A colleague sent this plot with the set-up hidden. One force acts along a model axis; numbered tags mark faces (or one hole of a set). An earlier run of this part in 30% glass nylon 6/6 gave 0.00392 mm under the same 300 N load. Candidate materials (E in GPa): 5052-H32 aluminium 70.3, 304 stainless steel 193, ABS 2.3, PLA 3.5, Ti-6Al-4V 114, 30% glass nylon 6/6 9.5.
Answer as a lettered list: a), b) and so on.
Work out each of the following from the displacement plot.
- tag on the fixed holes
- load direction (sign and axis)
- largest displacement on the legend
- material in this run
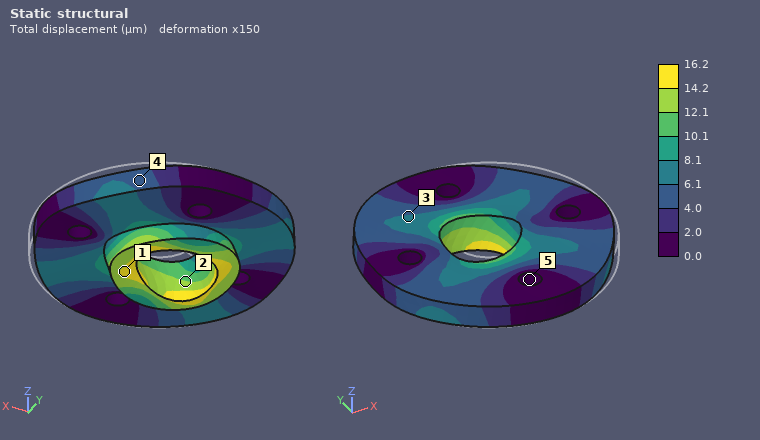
a) 5
b) -X
c) 16.2 µm
d) ABS
